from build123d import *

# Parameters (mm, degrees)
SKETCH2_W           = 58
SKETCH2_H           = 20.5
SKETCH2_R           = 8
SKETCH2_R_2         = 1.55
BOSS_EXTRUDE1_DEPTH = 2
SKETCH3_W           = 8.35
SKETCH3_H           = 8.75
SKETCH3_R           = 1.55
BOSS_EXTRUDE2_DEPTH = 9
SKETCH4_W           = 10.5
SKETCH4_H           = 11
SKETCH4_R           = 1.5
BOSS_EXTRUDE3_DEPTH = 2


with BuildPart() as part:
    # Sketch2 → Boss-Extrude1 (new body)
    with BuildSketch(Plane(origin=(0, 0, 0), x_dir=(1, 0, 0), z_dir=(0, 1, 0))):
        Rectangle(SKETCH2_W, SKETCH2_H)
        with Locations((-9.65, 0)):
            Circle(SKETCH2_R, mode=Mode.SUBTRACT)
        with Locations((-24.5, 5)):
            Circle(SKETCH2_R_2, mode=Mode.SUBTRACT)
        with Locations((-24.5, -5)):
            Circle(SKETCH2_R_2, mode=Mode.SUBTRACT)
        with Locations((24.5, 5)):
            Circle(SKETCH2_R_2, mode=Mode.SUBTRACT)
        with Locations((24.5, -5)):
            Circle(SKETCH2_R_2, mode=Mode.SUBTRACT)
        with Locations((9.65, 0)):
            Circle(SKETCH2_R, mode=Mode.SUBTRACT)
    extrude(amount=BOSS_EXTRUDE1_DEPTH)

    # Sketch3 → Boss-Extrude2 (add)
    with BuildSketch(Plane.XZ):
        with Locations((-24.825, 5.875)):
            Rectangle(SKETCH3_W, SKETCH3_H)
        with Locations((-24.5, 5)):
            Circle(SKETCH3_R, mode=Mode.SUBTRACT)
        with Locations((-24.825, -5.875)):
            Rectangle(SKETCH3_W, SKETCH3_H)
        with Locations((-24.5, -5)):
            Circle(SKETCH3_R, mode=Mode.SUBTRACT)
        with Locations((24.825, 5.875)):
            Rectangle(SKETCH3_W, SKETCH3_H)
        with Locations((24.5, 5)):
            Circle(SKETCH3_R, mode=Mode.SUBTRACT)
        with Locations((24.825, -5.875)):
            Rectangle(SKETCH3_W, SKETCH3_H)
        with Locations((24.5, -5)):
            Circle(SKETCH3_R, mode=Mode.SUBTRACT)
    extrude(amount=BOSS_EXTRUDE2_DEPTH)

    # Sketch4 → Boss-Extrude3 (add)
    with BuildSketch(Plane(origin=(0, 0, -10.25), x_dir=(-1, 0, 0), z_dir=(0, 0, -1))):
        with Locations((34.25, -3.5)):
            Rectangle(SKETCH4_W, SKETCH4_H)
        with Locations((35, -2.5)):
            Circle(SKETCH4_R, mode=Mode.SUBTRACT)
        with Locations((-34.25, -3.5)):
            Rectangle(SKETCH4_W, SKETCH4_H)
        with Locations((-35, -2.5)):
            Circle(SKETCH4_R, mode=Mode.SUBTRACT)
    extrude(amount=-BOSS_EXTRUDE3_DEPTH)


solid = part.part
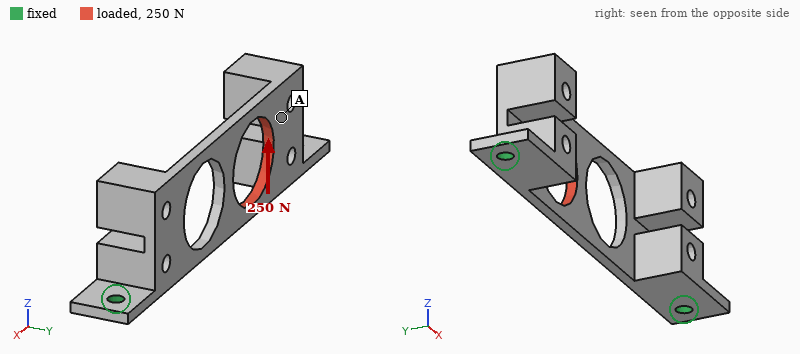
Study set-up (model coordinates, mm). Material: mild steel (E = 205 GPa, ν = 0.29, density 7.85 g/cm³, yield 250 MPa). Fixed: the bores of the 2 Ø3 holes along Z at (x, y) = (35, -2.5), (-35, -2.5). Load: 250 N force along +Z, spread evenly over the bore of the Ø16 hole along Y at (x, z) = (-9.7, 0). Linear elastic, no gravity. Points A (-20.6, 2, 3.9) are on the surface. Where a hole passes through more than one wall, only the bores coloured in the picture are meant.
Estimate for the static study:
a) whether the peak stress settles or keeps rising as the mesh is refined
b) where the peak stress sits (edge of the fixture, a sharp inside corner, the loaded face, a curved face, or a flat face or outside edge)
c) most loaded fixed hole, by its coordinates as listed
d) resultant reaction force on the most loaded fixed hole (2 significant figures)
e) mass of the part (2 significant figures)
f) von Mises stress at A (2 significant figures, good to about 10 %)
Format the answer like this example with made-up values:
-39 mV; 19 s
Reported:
keeps rising; edge of the fixture; (-35, -2.5); 190 N; 34 g; 17 MPa
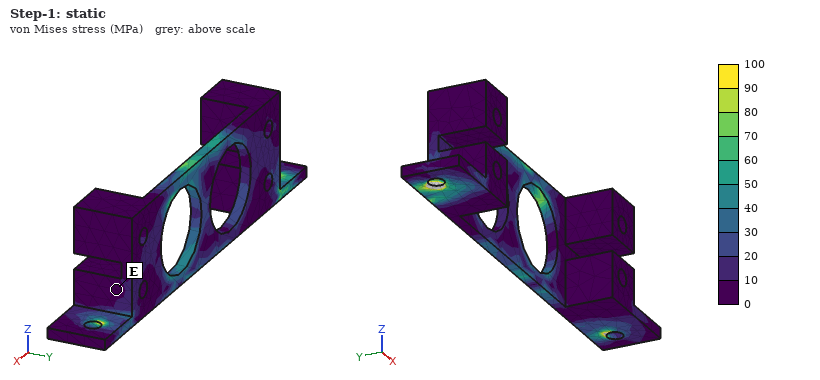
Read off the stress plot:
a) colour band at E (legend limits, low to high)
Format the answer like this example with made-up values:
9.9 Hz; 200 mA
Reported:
0 to 10 MPa
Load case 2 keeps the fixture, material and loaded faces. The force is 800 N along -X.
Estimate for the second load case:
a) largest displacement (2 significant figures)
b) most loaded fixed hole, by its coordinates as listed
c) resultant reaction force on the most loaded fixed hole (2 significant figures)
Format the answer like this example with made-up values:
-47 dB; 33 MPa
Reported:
25 µm; (-35, -2.5); 480 N
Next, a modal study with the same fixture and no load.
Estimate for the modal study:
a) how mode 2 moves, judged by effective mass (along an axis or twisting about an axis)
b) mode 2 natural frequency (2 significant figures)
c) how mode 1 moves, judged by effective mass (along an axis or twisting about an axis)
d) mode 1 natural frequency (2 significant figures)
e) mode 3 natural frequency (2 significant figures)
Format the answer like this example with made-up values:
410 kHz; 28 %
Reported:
twisting about Z; 2500 Hz; along Y; 2000 Hz; 4700 Hz
